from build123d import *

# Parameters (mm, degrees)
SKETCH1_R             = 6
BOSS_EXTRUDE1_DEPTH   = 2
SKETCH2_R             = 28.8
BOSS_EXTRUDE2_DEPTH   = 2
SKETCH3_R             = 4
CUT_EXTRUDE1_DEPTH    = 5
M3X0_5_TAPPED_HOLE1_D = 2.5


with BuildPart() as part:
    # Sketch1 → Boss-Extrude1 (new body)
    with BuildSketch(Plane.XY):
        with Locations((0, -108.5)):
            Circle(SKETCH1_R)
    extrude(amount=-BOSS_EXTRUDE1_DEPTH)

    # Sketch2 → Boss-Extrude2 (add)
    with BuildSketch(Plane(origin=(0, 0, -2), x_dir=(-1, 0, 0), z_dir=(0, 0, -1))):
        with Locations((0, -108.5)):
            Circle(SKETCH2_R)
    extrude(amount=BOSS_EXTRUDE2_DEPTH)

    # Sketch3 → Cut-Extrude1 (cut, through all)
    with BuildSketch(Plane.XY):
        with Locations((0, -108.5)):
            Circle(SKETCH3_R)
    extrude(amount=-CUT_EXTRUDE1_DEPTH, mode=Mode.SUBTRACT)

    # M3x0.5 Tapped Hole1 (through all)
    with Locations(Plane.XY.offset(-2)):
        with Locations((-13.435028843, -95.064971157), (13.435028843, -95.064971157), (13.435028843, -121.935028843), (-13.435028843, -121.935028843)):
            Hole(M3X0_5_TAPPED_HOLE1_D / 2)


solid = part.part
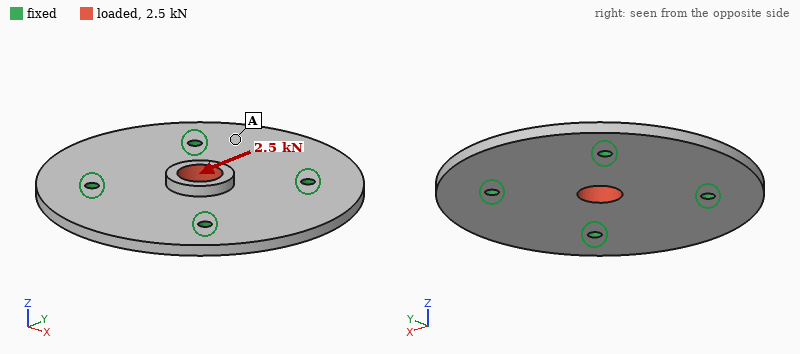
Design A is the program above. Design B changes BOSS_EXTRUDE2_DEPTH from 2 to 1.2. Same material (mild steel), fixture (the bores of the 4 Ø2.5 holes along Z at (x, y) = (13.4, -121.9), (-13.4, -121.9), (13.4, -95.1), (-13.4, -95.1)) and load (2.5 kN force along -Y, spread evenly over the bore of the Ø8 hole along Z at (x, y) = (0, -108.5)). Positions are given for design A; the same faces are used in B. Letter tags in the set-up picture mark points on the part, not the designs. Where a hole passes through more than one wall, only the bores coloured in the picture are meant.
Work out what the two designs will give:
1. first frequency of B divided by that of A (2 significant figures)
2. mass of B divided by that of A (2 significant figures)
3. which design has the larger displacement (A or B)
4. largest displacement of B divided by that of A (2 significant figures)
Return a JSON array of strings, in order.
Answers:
["0.63", "0.61", "B", "3.1"]
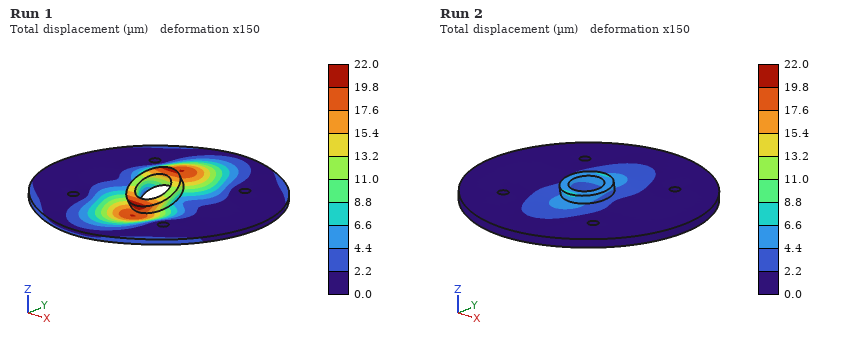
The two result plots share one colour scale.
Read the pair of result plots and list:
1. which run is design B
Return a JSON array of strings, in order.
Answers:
["Run 1"]
